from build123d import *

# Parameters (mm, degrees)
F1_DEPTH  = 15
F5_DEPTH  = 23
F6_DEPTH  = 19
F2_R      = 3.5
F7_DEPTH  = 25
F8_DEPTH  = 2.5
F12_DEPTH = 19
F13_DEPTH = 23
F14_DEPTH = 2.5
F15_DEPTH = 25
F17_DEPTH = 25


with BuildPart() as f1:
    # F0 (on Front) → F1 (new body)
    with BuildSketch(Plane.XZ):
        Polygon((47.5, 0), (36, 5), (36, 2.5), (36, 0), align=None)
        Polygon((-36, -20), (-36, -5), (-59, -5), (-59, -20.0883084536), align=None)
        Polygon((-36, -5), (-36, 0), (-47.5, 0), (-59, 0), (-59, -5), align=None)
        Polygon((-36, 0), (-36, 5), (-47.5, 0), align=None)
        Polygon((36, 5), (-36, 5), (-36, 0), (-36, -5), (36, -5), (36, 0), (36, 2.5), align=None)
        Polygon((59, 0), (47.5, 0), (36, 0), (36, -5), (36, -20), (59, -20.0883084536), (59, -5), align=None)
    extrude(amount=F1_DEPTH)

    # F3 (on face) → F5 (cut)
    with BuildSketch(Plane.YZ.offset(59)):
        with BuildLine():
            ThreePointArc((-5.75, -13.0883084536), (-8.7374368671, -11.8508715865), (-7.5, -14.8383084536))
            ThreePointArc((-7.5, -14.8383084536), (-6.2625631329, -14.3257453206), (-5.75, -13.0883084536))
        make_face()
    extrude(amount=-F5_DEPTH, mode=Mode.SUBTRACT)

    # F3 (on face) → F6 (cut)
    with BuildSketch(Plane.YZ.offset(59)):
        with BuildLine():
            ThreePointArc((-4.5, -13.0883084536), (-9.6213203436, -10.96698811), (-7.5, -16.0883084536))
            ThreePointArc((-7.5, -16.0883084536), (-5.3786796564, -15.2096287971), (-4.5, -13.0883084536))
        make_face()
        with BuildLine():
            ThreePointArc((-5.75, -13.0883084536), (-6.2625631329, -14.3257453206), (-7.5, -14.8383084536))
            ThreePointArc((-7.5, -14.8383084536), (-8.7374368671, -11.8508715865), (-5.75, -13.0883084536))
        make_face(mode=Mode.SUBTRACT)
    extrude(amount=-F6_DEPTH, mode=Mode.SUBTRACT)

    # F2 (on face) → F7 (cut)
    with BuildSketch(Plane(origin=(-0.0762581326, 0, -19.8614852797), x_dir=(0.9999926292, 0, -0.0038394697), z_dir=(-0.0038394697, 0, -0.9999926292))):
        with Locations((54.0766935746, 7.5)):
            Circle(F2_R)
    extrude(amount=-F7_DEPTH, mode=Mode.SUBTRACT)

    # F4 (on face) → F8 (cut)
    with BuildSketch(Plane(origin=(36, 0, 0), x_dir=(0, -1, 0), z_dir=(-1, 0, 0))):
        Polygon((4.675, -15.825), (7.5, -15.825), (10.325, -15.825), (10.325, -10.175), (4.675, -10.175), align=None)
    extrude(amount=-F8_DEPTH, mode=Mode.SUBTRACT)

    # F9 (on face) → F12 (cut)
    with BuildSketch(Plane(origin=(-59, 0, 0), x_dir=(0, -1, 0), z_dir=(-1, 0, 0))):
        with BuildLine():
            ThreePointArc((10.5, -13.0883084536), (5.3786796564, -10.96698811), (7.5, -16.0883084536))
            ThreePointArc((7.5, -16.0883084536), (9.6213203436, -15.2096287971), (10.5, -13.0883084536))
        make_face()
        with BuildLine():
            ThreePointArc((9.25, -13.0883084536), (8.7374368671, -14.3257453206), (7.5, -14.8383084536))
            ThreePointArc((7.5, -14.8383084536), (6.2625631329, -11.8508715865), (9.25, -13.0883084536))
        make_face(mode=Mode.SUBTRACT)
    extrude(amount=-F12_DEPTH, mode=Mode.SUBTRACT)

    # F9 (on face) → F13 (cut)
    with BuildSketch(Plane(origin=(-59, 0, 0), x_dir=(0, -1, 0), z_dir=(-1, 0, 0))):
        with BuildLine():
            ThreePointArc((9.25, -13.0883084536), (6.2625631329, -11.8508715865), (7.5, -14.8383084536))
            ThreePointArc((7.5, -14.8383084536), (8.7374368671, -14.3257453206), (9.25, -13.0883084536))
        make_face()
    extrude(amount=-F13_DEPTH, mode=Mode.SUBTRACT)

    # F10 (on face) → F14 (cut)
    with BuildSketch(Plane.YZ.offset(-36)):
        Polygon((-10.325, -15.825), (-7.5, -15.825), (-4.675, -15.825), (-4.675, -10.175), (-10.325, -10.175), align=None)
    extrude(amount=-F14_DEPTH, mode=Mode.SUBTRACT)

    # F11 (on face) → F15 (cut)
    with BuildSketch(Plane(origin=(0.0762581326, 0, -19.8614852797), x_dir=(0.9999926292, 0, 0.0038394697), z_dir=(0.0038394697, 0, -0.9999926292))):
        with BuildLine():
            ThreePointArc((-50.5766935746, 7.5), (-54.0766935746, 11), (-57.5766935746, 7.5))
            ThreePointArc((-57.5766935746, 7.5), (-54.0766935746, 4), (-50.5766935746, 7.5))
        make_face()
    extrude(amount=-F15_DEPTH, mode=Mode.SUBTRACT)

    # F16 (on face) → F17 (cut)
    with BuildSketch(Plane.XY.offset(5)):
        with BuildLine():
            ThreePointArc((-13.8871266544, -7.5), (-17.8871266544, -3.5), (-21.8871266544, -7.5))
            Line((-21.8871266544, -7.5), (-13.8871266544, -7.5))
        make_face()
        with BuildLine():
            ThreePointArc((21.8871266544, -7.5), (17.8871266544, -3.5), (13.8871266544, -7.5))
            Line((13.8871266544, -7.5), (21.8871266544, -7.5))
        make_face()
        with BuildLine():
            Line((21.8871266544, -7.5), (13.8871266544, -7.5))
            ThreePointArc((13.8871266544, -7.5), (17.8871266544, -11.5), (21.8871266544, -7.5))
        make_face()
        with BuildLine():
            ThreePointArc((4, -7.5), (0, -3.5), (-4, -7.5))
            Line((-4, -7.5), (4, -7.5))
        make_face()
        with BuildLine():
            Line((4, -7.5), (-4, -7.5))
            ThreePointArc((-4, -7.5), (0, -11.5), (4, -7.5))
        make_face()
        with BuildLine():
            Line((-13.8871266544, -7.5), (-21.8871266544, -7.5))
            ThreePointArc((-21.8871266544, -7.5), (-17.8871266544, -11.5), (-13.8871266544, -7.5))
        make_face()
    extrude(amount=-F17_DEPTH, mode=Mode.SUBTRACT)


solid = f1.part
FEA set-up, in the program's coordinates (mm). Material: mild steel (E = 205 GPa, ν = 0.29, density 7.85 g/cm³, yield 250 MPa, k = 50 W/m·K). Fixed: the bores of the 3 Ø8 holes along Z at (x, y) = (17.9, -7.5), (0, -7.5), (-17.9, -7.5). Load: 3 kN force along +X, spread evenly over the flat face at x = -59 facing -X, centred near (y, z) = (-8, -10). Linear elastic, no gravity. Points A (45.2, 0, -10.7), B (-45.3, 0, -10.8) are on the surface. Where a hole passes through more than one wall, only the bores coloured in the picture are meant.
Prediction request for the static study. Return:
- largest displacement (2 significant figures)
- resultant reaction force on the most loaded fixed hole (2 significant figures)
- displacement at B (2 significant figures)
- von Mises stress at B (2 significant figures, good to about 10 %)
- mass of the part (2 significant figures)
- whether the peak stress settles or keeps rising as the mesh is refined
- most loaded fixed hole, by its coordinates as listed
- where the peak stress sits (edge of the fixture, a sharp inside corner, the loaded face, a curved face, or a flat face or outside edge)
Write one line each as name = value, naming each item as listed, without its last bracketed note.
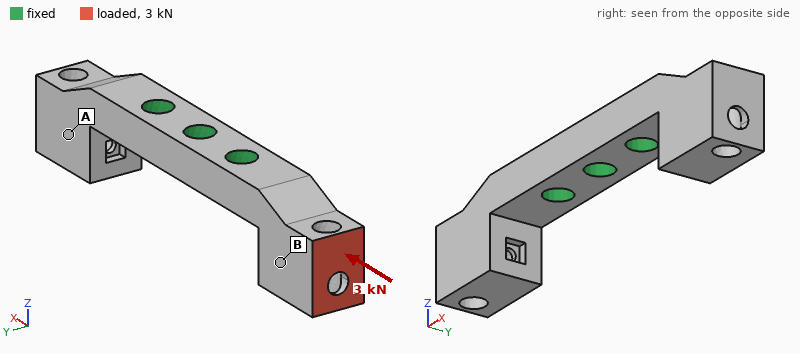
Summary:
largest displacement = 90 µm
resultant reaction force on the most loaded fixed hole = 2.9 kN
displacement at B = 46 µm
von Mises stress at B = 27 MPa
mass of the part = 170 g
whether the peak stress settles or keeps rising as the mesh is refined = keeps rising
most loaded fixed hole, by its coordinates as listed = (-17.9, -7.5)
where the peak stress sits = edge of the fixture
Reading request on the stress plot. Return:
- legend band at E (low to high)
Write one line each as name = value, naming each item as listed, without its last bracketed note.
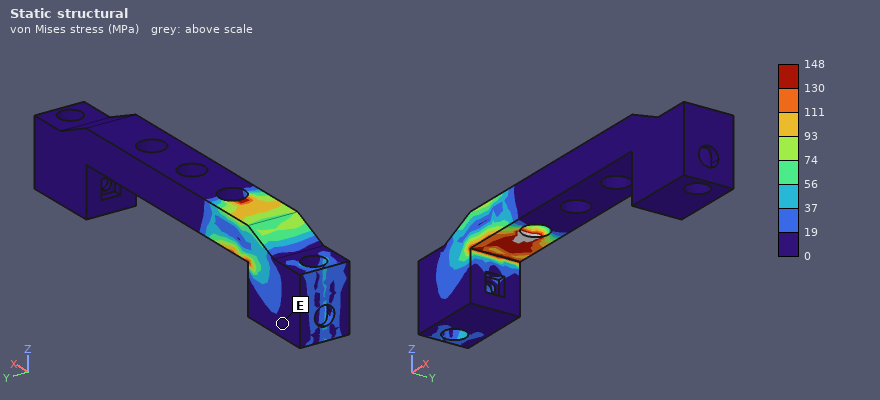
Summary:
legend band at E = 0 to 19 MPa
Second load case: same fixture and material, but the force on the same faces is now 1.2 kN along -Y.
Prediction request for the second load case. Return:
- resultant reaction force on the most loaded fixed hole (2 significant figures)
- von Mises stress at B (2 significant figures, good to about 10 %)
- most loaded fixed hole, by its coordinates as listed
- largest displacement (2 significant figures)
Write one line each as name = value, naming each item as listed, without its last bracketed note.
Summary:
resultant reaction force on the most loaded fixed hole = 1.6 kN
von Mises stress at B = 25 MPa
most loaded fixed hole, by its coordinates as listed = (-17.9, -7.5)
largest displacement = 74 µm
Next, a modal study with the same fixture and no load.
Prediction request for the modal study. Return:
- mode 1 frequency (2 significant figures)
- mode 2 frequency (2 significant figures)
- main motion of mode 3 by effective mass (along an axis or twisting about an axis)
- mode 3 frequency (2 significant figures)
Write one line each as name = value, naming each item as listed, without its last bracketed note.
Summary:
mode 1 frequency = 3700 Hz
mode 2 frequency = 3700 Hz
main motion of mode 3 by effective mass = along Y
mode 3 frequency = 4600 Hz
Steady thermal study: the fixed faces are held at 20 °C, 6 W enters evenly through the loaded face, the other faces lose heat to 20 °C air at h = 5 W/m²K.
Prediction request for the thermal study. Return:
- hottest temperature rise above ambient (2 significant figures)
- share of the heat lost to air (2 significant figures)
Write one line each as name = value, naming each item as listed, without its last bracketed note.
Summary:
hottest temperature rise above ambient = 29 K
share of the heat lost to air = 4.8 %
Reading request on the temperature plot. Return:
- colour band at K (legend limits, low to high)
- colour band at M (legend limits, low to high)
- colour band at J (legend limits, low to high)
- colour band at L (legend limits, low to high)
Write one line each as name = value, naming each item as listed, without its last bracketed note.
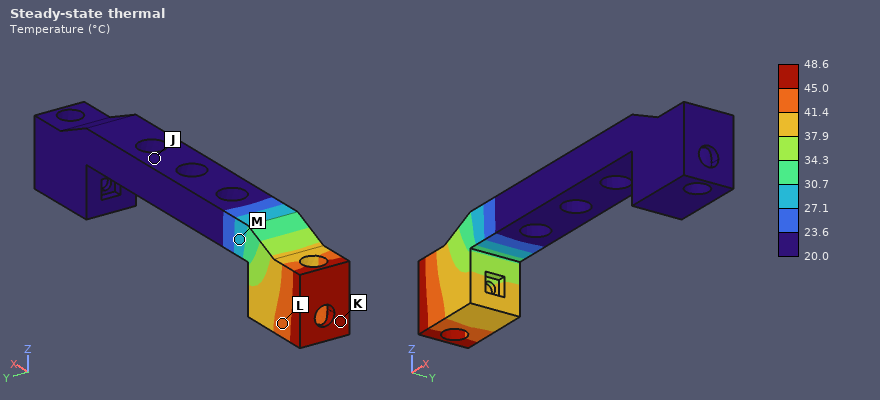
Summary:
colour band at K = 45.0 to 48.6 °C
colour band at M = 27.1 to 30.7 °C
colour band at J = 20.0 to 23.6 °C
colour band at L = 41.4 to 45.0 °C
